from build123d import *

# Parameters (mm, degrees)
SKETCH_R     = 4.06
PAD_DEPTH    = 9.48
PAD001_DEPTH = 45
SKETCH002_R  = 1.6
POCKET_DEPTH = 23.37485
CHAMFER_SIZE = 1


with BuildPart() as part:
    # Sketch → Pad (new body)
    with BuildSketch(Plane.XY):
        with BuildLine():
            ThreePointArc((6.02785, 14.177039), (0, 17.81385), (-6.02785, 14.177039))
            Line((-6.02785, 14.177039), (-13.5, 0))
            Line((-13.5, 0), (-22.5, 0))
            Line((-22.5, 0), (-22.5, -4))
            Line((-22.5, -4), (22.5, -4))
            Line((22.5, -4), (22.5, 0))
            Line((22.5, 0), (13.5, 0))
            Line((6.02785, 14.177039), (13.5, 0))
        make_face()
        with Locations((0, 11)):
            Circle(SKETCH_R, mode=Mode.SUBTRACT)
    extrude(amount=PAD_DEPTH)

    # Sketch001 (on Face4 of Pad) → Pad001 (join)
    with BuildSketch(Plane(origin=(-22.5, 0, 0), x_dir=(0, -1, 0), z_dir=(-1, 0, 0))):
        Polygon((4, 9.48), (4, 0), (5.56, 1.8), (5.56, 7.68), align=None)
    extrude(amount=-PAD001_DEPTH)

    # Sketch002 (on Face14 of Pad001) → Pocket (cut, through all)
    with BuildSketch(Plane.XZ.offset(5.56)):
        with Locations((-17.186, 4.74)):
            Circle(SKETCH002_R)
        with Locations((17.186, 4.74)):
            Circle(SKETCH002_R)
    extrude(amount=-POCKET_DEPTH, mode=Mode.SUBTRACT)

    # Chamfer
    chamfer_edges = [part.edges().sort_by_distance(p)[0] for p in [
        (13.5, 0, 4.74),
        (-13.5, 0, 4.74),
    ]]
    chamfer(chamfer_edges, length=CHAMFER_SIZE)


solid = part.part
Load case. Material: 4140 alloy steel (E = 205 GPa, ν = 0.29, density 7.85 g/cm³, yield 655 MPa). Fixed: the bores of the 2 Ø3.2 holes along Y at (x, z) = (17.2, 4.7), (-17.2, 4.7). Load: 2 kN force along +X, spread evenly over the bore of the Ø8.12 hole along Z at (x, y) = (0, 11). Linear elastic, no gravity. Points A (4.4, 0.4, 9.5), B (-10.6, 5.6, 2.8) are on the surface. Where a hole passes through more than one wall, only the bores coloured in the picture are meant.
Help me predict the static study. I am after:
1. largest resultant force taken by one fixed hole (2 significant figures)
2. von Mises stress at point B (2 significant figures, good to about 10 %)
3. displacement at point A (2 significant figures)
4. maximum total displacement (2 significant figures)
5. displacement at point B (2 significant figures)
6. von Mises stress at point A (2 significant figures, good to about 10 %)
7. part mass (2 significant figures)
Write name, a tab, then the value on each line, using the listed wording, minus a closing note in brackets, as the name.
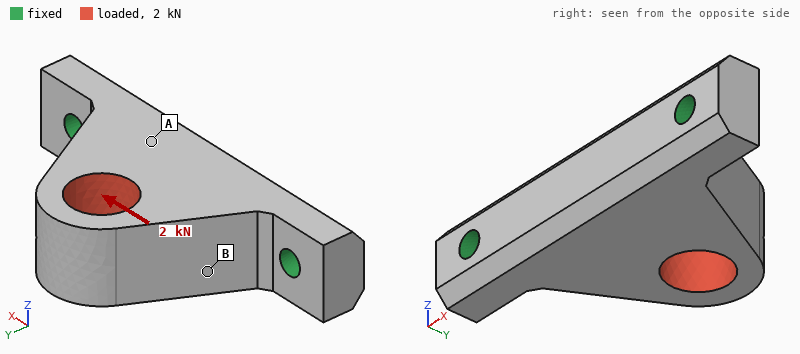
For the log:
largest resultant force taken by one fixed hole	1.4 kN
von Mises stress at point B	37 MPa
displacement at point A	1.2 µm
maximum total displacement	7.7 µm
displacement at point B	2.7 µm
von Mises stress at point A	10 MPa
part mass	36 g
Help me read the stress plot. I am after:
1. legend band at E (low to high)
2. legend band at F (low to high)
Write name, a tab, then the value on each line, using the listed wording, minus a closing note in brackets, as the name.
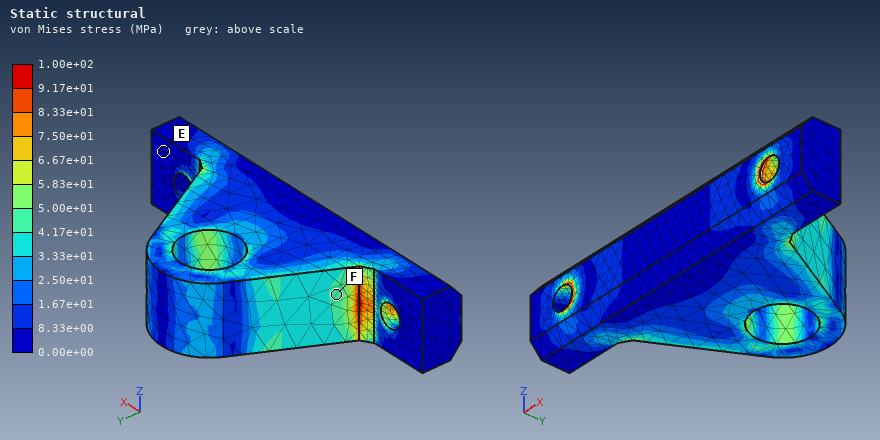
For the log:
legend band at E	0.00e+00 to 8.33e+00 MPa
legend band at F	4.17e+01 to 5.00e+01 MPa
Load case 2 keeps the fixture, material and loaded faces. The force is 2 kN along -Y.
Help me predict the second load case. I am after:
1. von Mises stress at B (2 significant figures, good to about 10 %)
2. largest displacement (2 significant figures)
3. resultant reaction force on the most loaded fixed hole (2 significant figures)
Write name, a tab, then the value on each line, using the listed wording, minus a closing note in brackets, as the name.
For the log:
von Mises stress at B	25 MPa
largest displacement	4.3 µm
resultant reaction force on the most loaded fixed hole	1.2 kN
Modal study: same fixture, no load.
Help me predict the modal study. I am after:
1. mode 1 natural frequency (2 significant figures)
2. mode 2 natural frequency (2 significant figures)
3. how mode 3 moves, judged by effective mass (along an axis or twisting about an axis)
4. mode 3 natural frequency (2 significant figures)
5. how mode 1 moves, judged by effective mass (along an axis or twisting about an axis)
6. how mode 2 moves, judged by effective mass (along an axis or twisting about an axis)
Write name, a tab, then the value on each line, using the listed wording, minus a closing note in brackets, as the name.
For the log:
mode 1 natural frequency	9500 Hz
mode 2 natural frequency	23 kHz
how mode 3 moves, judged by effective mass	along Z
mode 3 natural frequency	26 kHz
how mode 1 moves, judged by effective mass	along Z
how mode 2 moves, judged by effective mass	along Y
